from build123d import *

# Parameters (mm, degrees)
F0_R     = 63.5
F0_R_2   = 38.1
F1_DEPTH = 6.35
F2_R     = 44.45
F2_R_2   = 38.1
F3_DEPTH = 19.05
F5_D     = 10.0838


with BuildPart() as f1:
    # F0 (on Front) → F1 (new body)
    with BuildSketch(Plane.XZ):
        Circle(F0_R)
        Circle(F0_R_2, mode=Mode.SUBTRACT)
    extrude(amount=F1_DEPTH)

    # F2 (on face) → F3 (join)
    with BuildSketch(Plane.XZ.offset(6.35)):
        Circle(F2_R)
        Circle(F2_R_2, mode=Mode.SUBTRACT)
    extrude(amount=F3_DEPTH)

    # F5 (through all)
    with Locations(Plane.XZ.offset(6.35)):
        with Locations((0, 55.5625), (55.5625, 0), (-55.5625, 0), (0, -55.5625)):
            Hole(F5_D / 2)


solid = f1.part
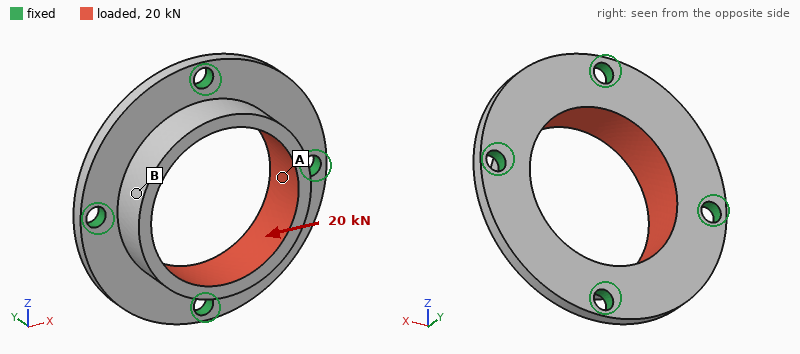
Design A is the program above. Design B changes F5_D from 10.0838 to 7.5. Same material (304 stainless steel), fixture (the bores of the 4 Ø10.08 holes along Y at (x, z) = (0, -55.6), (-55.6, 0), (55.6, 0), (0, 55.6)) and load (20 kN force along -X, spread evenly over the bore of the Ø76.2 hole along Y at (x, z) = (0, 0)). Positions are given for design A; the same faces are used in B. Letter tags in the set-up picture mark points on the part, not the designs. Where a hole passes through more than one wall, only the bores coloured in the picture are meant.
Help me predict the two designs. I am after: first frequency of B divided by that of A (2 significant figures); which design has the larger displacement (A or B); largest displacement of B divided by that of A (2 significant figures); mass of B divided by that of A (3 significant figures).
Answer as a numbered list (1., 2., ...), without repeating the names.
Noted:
1. 0.92
2. B
3. 1.1
4. 1.01
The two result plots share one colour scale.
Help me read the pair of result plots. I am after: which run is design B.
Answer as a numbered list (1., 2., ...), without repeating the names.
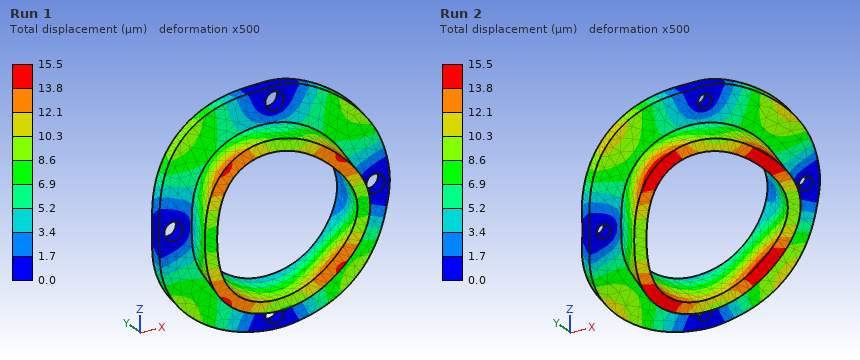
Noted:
1. Run 2
